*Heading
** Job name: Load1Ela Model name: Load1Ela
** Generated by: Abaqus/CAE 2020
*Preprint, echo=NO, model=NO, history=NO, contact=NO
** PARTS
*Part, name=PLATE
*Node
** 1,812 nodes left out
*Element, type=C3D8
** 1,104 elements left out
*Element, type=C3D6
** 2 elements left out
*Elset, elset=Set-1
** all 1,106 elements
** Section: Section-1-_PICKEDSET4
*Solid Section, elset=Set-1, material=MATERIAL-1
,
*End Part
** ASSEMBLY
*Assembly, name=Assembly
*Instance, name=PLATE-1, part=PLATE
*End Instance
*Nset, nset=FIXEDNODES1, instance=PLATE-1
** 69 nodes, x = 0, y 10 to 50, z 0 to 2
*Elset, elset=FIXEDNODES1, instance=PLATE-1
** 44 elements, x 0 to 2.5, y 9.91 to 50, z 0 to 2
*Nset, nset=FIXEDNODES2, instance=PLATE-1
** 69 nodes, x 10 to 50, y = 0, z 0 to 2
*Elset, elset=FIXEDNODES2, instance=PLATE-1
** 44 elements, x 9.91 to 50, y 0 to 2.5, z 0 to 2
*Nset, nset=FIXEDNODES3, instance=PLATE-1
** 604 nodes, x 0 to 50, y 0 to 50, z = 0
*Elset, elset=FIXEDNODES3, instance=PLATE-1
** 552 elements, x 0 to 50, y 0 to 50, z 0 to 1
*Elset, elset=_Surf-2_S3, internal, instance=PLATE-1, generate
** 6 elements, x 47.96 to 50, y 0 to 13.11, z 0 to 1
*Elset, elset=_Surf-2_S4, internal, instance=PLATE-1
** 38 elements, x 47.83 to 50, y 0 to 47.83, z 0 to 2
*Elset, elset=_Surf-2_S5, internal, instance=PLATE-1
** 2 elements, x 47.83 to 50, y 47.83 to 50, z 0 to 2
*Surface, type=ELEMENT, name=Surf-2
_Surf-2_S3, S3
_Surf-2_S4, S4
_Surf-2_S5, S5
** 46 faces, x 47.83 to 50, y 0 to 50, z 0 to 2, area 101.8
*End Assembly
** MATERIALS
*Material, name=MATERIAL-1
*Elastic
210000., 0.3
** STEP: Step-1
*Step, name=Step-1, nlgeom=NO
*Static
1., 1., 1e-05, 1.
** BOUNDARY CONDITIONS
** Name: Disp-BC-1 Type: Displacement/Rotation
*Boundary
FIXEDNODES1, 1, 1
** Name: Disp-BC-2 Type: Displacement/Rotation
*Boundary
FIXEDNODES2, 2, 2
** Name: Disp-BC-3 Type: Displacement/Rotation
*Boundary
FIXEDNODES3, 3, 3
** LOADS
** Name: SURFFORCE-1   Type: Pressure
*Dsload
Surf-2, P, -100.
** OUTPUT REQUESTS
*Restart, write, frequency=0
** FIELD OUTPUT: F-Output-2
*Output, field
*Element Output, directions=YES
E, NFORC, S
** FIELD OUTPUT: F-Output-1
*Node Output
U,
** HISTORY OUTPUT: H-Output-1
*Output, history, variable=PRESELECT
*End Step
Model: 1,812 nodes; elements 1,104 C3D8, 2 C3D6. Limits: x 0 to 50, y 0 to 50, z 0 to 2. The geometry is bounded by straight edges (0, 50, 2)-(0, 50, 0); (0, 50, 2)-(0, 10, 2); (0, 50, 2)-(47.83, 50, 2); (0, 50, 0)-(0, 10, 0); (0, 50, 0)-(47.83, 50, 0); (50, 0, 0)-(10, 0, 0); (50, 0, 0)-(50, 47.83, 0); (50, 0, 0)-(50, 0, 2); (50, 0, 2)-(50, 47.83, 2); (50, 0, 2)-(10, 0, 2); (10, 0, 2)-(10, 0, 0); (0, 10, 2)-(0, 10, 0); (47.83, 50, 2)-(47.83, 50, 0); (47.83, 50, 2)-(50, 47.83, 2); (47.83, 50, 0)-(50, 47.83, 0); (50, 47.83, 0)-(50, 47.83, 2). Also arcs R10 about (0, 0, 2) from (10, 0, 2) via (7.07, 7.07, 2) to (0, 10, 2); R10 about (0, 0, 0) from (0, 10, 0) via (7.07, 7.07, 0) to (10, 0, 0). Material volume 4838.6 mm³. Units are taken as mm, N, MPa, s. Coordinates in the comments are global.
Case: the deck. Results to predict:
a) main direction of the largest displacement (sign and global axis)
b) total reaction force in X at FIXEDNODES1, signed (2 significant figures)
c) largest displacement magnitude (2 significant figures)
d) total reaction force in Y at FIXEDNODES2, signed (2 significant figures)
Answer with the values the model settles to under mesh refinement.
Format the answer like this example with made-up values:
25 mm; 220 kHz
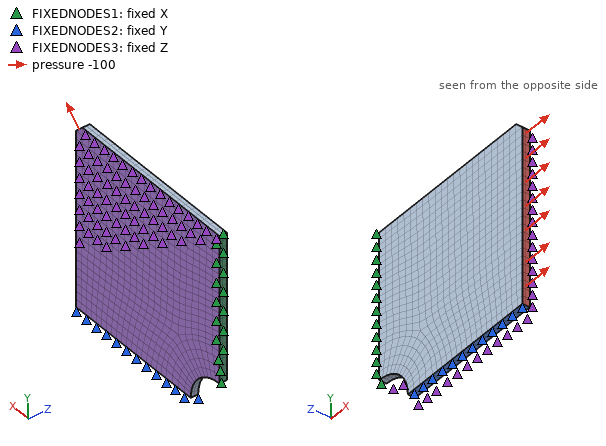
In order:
+X; -10000 N; 0.030 mm; -430 N
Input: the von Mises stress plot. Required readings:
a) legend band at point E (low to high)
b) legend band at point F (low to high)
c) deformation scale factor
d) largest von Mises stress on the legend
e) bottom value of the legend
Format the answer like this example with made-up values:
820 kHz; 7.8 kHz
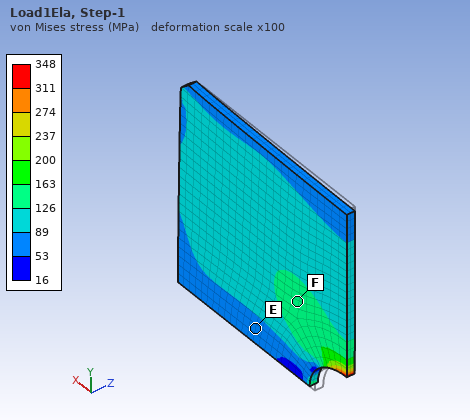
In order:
53 to 89 MPa; 126 to 163 MPa; 100; 348 MPa; 16 MPa
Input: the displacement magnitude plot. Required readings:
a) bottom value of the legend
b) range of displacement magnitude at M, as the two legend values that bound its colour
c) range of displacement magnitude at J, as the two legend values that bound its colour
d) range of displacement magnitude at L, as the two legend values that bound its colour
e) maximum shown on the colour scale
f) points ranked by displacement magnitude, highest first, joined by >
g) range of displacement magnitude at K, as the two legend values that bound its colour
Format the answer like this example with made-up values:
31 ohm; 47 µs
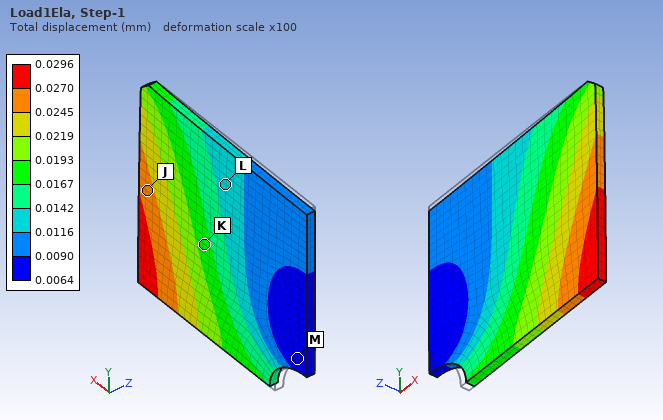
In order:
0.0064 mm; 0.0064 to 0.0090 mm; 0.0245 to 0.0270 mm; 0.0116 to 0.0142 mm; 0.0296 mm; J > K > L > M; 0.0167 to 0.0193 mm
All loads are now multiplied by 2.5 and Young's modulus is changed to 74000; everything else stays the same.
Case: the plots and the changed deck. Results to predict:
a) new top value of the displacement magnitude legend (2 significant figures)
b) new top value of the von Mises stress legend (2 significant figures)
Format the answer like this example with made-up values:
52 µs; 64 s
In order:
0.21 mm; 870 MPa
